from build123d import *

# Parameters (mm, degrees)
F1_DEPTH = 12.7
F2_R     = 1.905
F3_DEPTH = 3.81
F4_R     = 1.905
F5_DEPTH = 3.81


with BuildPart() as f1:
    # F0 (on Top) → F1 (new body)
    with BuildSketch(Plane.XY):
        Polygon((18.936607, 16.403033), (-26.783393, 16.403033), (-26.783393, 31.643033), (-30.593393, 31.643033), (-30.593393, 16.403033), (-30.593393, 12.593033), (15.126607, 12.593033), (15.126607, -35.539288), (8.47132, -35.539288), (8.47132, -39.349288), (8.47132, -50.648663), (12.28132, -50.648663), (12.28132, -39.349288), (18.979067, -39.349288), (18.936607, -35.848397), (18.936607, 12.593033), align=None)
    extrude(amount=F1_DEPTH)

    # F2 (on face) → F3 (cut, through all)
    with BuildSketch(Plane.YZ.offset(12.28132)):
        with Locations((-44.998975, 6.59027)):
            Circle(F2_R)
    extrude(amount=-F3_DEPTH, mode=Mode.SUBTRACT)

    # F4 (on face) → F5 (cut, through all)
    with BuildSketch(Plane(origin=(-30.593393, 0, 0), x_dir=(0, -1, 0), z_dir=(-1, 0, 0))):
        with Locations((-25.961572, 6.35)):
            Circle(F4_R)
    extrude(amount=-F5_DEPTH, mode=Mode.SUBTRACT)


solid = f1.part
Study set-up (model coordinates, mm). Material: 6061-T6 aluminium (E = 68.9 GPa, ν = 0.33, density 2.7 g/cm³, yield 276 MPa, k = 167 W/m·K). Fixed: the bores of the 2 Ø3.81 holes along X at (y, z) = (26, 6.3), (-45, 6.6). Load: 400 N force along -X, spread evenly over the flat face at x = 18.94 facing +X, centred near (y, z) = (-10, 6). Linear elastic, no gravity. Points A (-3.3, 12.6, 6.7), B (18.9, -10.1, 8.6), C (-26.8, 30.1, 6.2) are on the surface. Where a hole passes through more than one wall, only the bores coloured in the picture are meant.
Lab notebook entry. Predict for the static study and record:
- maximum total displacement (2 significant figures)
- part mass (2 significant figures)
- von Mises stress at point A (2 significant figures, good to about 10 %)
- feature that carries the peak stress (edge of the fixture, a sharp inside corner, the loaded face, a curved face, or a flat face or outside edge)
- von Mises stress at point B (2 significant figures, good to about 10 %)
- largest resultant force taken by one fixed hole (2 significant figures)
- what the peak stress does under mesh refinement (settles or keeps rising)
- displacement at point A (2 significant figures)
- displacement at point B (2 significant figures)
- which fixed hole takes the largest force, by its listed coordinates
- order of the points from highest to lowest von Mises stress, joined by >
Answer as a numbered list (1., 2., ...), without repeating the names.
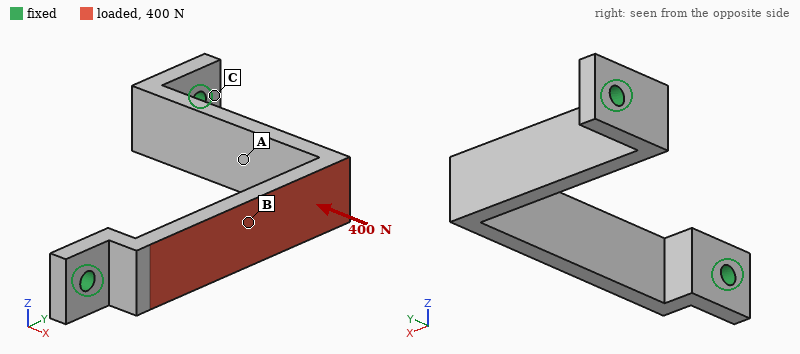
1. 89 µm
2. 17 g
3. 15 MPa
4. edge of the fixture
5. 42 MPa
6. 230 N
7. keeps rising
8. 27 µm
9. 86 µm
10. (26, 6.3)
11. B > A > C
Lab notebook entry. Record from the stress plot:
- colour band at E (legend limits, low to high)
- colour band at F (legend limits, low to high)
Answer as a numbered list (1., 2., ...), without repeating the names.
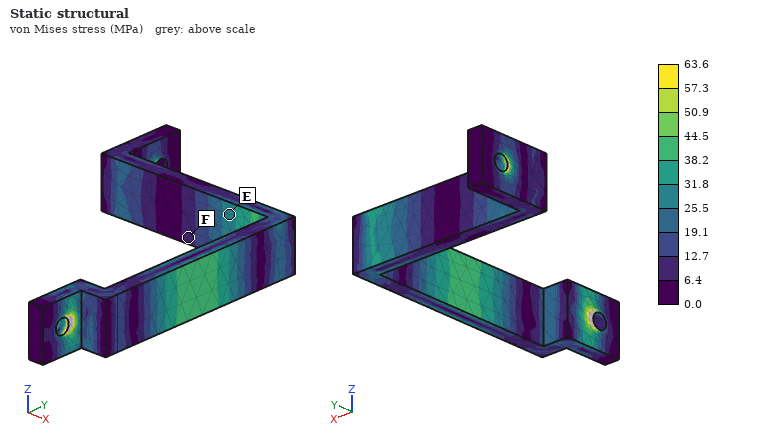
1. 25.5 to 31.8 MPa
2. 6.4 to 12.7 MPa
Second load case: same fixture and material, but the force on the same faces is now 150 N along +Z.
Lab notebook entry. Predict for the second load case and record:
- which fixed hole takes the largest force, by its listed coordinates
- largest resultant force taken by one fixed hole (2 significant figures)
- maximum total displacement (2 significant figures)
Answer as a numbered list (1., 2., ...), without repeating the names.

1. (-45, 6.6)
2. 120 N
3. 0.14 mm
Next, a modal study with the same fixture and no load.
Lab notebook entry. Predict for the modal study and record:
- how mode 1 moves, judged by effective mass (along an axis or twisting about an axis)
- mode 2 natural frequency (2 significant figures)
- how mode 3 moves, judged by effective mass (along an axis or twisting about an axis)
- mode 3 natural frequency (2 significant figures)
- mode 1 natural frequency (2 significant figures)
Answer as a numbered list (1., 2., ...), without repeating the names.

1. along Z
2. 4000 Hz
3. along X
4. 5200 Hz
5. 1900 Hz
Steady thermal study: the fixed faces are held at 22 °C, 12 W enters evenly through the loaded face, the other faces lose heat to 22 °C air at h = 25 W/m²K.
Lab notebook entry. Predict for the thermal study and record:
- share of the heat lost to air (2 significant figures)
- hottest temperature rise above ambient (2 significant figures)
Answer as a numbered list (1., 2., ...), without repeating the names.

1. 10 %
2. 27 K
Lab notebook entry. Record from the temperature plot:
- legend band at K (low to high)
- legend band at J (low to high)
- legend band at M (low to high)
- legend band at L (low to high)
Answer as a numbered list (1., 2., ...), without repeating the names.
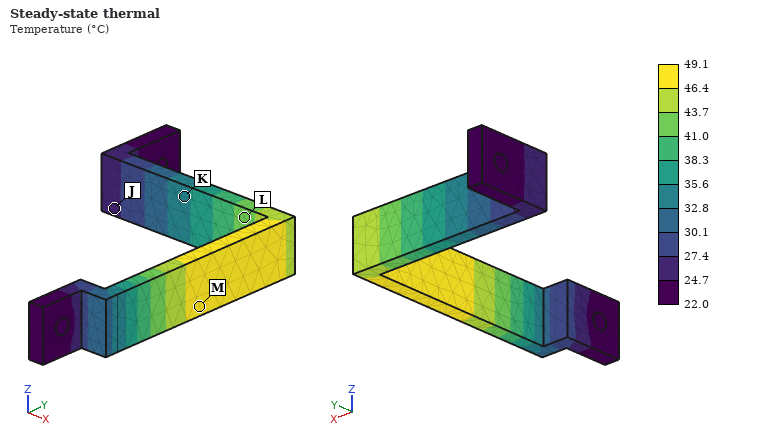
1. 32.8 to 35.6 °C
2. 24.7 to 27.4 °C
3. 46.4 to 49.1 °C
4. 41.0 to 43.7 °C
